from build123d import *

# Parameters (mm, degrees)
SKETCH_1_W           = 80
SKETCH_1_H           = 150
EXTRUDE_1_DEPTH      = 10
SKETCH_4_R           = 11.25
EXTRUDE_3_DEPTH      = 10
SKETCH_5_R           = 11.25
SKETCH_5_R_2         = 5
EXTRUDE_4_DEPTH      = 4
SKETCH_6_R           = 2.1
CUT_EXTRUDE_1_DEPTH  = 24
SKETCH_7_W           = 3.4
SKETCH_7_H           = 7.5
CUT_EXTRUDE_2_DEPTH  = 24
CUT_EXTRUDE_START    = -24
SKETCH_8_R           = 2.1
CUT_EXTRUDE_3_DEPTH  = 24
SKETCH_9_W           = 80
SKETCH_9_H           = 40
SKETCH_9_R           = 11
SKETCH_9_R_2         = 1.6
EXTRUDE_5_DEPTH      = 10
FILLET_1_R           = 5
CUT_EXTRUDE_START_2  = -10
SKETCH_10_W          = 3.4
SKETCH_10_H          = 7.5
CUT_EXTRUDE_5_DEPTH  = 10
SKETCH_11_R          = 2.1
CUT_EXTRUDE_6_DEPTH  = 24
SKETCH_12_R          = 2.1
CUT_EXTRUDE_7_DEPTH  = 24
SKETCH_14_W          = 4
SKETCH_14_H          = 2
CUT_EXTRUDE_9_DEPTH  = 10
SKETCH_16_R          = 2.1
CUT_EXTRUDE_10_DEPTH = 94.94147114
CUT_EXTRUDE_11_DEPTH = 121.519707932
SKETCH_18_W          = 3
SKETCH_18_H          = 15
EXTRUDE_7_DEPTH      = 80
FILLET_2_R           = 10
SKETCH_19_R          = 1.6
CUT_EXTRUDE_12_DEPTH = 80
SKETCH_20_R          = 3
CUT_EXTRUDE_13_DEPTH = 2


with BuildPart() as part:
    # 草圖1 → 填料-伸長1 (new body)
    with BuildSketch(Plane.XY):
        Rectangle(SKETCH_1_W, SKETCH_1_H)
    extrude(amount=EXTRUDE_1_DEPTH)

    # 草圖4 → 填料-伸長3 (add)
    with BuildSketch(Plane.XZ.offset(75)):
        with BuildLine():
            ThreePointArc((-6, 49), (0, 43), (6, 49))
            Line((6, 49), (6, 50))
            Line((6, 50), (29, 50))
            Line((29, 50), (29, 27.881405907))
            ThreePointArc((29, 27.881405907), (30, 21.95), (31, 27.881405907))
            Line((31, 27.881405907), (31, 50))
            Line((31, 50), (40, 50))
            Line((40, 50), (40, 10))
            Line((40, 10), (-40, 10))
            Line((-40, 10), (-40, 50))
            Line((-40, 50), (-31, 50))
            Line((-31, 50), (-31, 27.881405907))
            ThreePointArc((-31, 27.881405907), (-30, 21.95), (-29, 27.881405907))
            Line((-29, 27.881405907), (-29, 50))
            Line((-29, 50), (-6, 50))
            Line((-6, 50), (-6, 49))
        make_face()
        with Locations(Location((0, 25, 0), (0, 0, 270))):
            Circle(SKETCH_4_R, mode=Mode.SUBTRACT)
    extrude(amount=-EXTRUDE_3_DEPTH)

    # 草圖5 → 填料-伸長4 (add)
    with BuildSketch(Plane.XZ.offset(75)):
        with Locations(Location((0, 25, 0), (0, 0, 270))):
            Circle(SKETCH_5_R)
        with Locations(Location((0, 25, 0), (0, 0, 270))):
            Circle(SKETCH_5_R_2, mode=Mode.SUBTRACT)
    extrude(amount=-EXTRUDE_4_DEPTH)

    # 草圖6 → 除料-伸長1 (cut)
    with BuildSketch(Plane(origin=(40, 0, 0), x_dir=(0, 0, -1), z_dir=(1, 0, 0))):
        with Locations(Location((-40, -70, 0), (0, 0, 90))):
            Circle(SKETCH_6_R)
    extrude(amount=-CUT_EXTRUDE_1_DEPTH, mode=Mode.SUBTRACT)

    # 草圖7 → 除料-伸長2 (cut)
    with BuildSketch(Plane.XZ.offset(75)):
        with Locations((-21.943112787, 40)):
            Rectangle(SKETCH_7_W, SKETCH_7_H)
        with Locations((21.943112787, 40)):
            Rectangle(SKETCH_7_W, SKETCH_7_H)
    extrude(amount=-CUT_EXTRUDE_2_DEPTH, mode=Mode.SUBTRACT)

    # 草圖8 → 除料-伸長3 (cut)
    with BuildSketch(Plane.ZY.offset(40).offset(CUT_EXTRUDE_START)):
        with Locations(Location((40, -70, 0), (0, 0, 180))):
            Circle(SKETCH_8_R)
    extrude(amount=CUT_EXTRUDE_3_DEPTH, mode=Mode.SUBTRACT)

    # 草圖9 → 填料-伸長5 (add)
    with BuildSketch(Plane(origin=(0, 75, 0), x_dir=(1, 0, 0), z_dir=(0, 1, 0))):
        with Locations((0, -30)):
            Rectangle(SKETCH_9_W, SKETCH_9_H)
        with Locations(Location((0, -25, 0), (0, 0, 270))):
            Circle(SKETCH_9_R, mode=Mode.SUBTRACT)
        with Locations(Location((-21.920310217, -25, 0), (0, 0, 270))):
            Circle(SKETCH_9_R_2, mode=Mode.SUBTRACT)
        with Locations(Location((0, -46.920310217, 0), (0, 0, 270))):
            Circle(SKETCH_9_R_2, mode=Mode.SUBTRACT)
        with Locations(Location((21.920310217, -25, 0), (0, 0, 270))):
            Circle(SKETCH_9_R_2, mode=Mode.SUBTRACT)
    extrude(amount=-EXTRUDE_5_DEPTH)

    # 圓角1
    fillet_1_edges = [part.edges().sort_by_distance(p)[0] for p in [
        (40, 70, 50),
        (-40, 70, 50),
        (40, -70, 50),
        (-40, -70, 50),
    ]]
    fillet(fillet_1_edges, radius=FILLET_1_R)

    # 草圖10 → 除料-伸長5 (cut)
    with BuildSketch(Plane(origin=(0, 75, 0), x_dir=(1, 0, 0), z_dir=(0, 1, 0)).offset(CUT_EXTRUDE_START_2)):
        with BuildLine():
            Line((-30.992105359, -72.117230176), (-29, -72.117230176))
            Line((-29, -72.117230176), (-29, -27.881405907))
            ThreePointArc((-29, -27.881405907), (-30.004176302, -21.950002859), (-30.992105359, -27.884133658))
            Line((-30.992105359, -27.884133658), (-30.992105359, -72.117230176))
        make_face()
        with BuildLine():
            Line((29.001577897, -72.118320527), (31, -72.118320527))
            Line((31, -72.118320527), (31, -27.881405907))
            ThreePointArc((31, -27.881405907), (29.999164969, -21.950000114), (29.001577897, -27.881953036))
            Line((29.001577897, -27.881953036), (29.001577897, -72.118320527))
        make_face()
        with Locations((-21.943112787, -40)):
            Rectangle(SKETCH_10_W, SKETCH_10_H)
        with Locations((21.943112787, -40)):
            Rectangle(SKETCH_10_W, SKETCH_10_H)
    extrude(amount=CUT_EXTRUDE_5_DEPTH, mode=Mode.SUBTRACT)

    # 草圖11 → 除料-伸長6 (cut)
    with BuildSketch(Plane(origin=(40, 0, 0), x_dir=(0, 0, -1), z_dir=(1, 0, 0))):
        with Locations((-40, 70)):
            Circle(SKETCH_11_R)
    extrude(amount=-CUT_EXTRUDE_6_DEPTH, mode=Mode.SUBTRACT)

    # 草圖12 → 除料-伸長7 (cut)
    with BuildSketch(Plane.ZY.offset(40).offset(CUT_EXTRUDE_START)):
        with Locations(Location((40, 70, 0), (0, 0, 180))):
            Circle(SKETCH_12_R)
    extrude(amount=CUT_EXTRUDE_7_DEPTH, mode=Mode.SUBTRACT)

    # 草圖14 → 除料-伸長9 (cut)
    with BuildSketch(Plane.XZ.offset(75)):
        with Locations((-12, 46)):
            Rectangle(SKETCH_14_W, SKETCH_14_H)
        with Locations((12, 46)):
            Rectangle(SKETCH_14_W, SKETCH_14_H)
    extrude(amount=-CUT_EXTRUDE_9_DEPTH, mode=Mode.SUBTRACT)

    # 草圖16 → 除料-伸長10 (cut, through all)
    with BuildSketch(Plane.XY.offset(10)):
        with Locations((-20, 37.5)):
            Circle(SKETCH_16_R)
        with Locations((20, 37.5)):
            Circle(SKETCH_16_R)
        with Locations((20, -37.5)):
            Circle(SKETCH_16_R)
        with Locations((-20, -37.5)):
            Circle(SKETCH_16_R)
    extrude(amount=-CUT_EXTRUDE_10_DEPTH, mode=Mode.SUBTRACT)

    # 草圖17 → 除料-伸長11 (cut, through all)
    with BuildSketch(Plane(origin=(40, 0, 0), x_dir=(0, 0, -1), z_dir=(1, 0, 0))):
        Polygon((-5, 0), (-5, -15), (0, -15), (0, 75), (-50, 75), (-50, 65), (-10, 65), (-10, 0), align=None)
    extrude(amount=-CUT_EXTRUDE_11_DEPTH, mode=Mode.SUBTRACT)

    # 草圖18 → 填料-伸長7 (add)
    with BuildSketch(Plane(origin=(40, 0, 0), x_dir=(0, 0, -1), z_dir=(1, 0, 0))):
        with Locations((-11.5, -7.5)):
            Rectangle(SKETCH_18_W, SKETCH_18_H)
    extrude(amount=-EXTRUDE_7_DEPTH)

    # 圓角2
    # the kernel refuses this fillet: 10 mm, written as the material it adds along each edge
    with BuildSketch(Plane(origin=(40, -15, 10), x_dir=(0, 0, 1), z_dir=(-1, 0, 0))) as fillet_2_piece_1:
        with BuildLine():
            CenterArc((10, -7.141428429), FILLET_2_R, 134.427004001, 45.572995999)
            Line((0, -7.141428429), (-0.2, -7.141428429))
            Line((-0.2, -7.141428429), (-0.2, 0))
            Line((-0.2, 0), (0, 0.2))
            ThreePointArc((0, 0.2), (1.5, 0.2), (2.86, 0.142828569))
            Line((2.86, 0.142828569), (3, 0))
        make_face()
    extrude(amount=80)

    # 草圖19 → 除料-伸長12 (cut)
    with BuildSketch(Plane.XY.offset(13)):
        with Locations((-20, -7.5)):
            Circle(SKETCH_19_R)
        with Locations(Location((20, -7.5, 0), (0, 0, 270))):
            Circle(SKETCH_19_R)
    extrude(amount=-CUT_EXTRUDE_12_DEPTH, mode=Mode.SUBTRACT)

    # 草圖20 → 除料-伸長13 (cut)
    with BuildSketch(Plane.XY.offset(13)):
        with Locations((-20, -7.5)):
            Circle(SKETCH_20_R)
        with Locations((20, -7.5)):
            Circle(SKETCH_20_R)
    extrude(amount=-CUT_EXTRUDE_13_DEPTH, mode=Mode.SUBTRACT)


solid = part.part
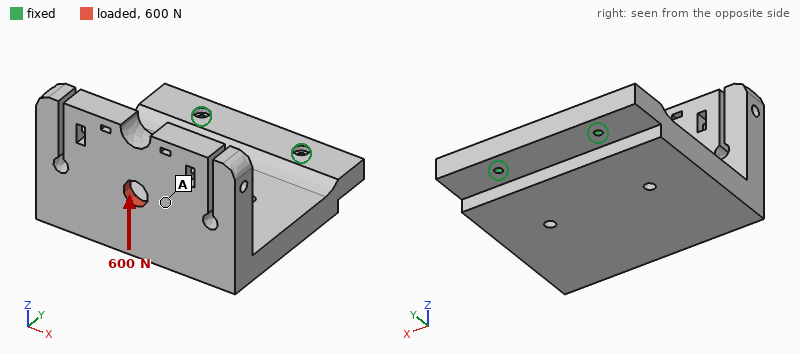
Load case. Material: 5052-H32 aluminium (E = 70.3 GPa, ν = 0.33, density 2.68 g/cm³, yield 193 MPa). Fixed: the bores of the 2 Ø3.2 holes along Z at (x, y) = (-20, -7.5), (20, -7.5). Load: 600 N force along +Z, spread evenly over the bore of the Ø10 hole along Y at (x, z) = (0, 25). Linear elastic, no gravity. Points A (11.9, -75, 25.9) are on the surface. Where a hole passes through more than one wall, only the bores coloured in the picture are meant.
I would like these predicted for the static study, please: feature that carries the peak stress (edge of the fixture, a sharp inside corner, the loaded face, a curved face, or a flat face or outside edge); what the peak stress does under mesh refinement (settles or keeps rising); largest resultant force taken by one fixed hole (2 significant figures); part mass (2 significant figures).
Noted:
edge of the fixture
keeps rising
300 N
220 g
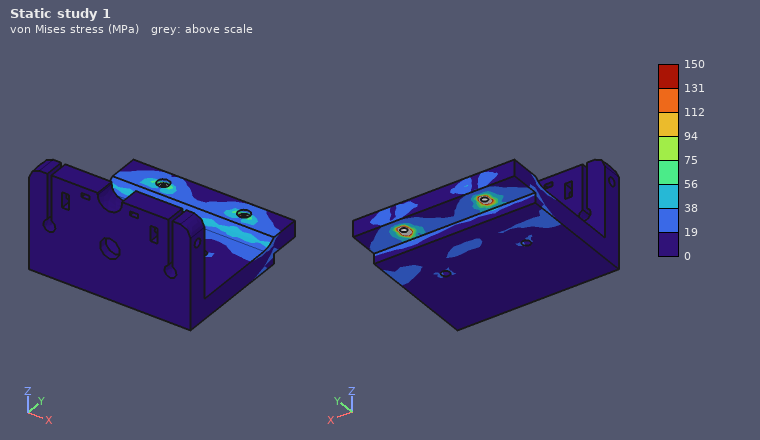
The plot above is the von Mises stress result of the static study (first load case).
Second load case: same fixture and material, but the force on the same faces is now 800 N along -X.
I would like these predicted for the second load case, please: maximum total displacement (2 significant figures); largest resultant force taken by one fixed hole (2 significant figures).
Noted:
0.10 mm
1.4 kN
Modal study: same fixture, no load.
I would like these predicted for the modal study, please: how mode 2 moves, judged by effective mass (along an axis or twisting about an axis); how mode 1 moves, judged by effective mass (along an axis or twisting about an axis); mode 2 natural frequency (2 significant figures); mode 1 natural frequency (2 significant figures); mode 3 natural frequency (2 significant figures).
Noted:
along X
along Z
1400 Hz
590 Hz
2700 Hz
